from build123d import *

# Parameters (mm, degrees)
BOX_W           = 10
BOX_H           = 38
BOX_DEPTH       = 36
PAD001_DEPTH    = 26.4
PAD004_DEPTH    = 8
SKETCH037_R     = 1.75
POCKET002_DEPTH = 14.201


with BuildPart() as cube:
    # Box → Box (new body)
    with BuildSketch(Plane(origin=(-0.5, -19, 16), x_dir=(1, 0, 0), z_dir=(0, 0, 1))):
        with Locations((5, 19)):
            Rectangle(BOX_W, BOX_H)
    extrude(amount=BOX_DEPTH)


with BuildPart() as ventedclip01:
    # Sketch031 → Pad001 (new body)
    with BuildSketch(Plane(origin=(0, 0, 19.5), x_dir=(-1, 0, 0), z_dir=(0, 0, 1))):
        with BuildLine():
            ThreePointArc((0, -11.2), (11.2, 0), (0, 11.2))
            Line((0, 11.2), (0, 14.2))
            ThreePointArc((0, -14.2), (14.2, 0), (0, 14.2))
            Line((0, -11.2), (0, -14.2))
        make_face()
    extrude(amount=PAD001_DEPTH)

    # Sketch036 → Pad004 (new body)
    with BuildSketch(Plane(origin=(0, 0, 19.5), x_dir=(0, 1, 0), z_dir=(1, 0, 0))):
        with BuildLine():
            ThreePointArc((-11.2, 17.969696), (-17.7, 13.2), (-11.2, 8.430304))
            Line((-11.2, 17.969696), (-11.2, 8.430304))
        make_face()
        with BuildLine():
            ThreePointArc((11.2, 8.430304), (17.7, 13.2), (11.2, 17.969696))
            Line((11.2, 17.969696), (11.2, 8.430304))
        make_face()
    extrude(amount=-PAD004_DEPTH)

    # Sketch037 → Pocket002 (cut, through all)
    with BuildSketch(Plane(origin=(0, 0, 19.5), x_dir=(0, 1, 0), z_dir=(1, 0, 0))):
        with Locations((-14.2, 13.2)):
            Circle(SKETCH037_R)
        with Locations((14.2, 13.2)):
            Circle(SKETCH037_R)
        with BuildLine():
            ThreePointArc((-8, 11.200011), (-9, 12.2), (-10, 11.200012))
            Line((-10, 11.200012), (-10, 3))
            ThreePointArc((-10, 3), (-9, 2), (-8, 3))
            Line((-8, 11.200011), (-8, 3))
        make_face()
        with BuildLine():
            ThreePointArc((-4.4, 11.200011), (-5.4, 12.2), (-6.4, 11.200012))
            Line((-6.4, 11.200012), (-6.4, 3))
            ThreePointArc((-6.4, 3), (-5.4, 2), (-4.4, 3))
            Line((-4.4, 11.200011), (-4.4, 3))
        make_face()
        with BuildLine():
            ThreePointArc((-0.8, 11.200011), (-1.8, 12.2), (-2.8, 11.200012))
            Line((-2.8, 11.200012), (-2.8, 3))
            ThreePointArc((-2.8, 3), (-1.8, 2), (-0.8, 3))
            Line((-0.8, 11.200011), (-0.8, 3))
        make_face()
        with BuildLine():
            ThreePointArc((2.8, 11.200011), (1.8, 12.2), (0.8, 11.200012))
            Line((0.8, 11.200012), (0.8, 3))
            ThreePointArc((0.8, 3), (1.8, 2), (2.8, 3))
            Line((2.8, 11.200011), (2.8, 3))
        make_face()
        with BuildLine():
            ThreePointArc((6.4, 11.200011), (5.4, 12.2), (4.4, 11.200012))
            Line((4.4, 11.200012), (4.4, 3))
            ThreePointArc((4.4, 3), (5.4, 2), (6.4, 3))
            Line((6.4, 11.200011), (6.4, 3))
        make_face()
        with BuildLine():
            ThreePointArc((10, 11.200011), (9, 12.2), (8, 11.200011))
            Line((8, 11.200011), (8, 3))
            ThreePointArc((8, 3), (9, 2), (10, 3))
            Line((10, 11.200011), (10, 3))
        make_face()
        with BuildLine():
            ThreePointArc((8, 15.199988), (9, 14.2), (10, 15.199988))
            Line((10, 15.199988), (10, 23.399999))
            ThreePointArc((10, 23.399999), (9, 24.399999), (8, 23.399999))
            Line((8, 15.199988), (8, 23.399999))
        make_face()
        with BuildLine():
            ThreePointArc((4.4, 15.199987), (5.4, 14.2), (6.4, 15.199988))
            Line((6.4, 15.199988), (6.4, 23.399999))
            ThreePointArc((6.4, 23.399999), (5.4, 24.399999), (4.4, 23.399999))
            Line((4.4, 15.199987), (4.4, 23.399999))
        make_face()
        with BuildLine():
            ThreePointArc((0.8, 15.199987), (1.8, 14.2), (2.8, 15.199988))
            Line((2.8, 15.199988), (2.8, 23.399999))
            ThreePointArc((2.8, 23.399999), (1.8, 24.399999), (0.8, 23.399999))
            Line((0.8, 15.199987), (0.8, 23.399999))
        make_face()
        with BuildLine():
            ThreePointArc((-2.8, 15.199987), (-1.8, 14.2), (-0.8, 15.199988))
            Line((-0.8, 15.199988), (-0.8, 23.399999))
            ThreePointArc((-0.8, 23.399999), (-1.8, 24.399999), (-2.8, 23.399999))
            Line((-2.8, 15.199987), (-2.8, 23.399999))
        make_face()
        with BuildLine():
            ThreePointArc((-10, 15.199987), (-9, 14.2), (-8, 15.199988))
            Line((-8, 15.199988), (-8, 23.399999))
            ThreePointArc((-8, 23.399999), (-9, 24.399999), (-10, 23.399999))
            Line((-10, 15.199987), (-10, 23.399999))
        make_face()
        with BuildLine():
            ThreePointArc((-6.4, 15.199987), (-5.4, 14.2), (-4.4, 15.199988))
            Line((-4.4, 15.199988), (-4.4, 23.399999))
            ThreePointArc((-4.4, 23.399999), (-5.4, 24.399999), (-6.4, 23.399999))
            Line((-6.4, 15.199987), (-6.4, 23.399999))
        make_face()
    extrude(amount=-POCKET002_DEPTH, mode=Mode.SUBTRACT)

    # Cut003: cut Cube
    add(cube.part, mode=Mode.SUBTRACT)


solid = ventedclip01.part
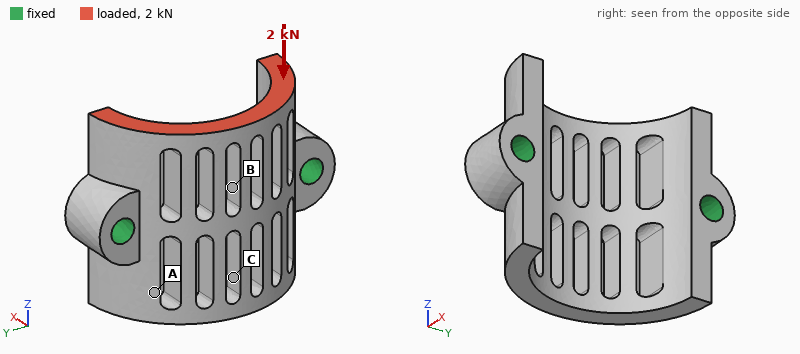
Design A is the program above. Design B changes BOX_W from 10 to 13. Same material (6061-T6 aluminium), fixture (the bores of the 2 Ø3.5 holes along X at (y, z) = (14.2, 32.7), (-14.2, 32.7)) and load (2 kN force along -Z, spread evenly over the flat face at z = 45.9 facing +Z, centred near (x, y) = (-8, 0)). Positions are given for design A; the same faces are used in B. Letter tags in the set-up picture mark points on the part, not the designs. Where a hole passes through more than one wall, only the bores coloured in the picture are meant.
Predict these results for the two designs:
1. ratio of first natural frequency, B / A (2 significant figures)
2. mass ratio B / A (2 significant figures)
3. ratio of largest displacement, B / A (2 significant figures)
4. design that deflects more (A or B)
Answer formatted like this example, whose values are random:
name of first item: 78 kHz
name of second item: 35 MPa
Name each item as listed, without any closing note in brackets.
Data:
ratio of first natural frequency, B / A: 0.92
mass ratio B / A: 0.89
ratio of largest displacement, B / A: 1.2
design that deflects more: B
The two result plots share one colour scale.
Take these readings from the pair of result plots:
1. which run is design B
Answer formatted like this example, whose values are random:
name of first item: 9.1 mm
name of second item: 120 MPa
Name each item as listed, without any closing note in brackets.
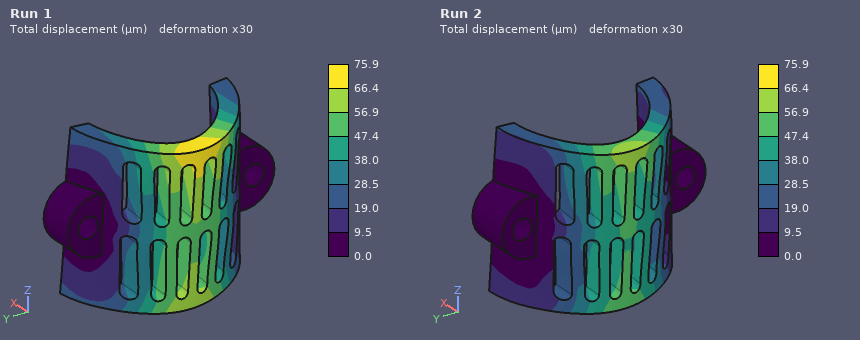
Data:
which run is design B: Run 1
